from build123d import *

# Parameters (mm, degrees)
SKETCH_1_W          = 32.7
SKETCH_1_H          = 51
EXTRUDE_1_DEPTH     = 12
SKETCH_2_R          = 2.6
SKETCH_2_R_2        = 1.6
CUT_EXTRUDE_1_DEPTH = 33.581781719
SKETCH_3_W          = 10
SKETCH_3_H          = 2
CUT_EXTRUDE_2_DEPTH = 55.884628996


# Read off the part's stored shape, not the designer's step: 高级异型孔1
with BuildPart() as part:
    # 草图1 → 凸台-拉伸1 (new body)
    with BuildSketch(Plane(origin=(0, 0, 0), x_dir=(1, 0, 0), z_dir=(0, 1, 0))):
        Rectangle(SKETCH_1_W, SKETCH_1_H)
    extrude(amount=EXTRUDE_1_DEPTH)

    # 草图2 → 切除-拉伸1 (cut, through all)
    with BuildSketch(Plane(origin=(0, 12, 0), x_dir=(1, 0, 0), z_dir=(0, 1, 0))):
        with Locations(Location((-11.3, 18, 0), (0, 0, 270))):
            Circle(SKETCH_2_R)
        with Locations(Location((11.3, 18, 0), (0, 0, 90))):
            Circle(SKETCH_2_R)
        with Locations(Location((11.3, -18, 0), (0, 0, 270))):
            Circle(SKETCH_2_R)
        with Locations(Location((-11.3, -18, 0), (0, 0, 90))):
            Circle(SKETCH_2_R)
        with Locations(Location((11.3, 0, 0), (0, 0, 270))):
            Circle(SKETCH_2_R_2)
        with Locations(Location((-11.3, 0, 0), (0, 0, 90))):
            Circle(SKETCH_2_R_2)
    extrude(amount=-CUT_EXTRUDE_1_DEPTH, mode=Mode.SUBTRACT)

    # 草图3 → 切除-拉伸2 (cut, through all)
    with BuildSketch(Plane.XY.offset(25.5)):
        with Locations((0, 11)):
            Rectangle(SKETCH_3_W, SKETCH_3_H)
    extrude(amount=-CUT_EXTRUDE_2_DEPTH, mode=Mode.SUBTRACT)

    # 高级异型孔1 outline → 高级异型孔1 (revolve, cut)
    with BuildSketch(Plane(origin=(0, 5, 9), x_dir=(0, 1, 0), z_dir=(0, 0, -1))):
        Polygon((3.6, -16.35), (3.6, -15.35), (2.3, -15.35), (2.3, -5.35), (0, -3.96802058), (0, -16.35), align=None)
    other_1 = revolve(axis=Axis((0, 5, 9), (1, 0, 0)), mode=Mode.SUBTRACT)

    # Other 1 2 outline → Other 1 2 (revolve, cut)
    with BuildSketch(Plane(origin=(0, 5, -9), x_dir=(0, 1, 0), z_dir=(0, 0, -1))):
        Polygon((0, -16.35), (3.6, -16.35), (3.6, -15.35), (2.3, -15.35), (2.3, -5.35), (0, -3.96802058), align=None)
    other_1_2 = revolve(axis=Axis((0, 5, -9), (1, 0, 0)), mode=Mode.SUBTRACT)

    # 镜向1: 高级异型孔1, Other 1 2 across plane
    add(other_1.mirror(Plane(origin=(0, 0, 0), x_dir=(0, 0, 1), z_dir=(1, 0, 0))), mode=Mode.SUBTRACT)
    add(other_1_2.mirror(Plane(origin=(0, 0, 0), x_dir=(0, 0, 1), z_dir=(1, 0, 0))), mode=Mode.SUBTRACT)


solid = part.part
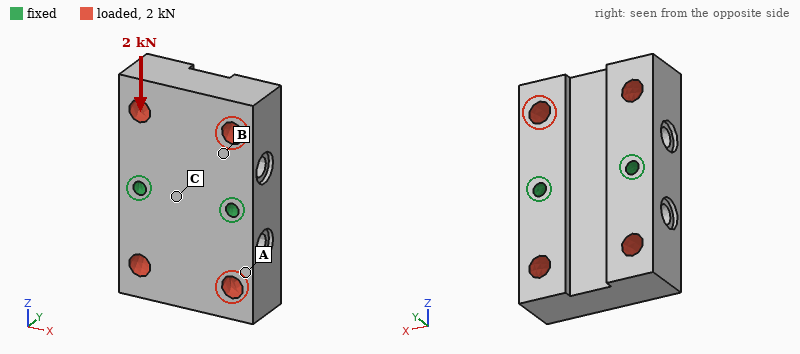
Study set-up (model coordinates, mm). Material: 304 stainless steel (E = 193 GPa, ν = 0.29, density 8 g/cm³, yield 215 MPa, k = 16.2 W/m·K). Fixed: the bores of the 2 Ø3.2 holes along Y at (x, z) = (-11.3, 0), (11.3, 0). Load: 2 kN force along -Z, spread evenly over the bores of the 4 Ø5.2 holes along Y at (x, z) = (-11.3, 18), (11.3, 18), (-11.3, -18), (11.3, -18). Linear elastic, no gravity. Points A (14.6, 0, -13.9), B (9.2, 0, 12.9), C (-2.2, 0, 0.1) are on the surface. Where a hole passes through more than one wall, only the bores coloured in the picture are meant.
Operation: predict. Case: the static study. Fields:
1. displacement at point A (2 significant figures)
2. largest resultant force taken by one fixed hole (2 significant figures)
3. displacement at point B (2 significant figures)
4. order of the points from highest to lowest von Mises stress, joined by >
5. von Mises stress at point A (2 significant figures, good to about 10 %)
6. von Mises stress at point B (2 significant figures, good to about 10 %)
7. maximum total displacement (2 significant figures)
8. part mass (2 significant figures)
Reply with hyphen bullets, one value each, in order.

- 0.42 µm
- 1.0 kN
- 0.33 µm
- A > B > C
- 6.2 MPa
- 3.9 MPa
- 0.60 µm
- 140 g
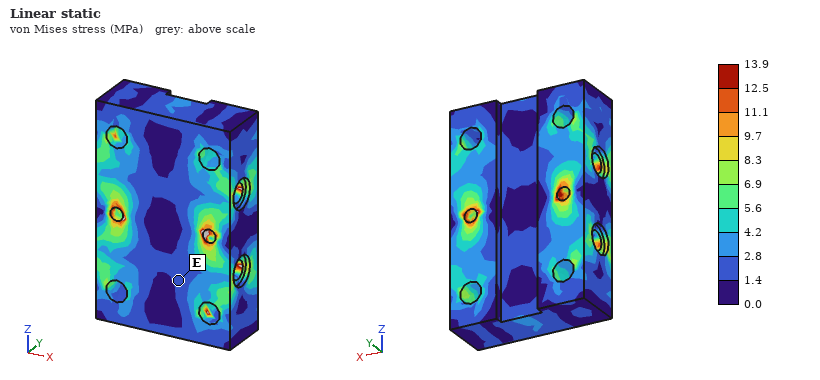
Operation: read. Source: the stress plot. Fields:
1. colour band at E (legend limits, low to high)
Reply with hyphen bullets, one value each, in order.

- 1.4 to 2.8 MPa
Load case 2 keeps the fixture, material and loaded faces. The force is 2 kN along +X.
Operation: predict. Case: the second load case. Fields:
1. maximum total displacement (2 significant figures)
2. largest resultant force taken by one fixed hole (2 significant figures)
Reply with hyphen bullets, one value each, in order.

- 1.8 µm
- 1.0 kN
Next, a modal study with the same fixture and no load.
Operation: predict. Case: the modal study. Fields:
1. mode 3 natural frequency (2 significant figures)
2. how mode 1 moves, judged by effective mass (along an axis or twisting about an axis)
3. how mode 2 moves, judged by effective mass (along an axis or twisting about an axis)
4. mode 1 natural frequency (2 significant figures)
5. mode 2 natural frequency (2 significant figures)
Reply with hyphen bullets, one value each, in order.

- 18 kHz
- twisting about X
- along Y
- 10 kHz
- 12 kHz
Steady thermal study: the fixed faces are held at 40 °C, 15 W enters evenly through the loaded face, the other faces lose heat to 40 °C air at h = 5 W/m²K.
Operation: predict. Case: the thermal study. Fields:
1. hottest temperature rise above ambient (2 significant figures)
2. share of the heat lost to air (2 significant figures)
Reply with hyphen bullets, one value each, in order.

- 34 K
- 4.2 %
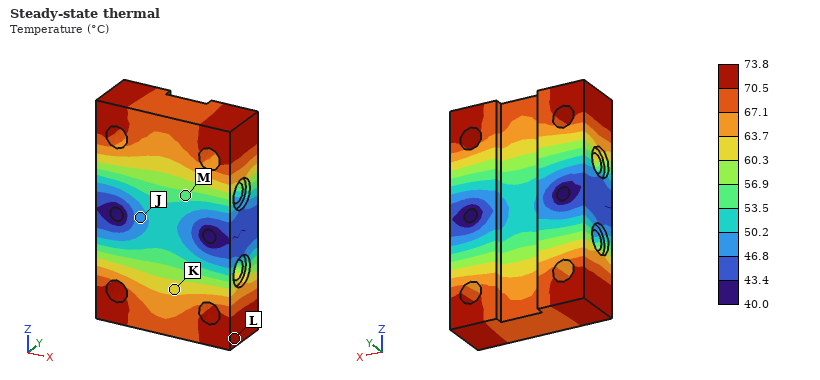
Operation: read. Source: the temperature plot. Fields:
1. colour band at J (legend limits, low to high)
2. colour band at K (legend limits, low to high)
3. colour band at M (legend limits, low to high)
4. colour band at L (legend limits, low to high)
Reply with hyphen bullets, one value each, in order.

- 46.8 to 50.2 °C
- 60.3 to 63.7 °C
- 53.5 to 56.9 °C
- 70.5 to 73.8 °C
